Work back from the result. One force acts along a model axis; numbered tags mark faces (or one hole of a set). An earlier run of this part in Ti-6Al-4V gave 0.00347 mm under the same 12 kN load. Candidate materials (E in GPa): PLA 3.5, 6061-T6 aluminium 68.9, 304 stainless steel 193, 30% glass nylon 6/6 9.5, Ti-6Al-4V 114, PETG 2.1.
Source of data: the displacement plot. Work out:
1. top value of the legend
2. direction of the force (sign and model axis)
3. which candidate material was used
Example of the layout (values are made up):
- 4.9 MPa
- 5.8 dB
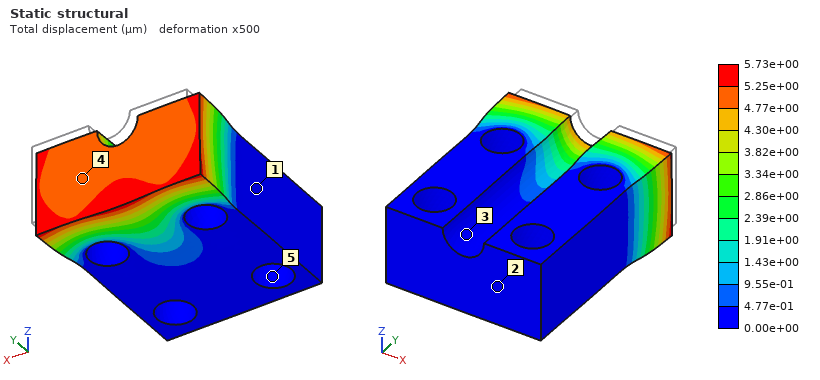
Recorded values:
- 5.73e+00 µm
- -Y
- 6061-T6 aluminium
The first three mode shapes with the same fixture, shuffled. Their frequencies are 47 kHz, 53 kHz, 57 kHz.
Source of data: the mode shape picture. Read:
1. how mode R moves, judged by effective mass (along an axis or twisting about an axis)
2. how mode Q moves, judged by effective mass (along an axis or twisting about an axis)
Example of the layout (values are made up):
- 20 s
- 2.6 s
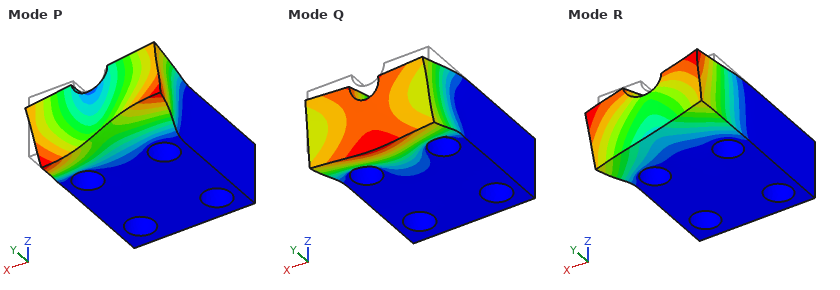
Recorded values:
- along X
- along Z
